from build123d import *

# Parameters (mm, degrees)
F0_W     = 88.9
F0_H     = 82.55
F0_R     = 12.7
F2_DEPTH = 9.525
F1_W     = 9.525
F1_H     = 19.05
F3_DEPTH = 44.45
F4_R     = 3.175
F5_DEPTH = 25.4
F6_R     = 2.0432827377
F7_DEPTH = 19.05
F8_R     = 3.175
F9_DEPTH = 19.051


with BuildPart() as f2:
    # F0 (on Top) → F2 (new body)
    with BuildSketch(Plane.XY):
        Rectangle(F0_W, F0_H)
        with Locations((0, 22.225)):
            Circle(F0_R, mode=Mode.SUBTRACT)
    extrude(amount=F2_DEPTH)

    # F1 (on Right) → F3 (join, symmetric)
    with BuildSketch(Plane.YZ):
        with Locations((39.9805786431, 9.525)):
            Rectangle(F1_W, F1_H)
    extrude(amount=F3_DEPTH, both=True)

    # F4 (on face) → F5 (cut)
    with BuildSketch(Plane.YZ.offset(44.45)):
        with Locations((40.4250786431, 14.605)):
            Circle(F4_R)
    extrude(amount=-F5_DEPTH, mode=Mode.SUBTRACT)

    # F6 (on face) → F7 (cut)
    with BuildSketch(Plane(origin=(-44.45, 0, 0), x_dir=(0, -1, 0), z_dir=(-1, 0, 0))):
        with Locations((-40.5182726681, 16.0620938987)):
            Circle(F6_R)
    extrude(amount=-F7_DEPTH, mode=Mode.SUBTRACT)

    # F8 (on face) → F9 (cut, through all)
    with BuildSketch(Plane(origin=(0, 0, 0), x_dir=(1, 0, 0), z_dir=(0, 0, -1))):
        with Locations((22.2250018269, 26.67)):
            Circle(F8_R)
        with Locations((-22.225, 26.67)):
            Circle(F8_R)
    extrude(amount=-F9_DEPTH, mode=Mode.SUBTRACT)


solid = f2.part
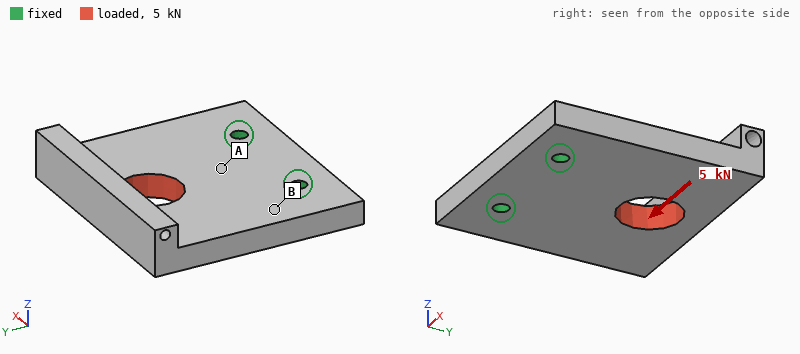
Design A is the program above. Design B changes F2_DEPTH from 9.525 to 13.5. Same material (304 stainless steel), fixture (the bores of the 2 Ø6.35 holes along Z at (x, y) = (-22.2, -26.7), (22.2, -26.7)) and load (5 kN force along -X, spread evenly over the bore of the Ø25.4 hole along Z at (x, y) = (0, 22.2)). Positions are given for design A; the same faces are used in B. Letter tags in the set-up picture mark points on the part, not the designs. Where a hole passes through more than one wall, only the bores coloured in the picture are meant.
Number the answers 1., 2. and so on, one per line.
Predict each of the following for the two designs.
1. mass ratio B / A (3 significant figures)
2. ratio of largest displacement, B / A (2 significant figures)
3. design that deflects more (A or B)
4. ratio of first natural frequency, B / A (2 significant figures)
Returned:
1. 1.33
2. 0.71
3. A
4. 1.5
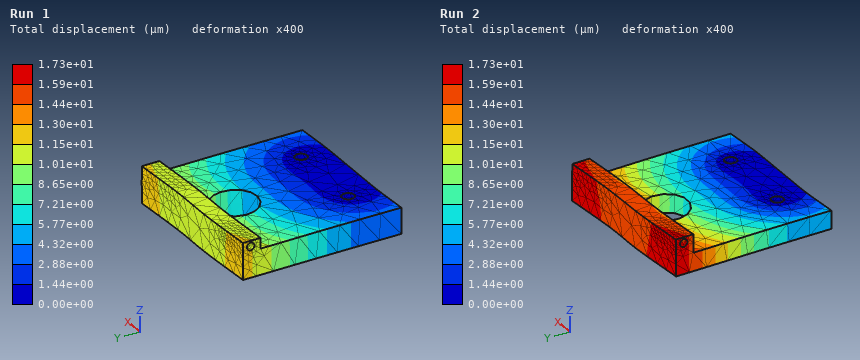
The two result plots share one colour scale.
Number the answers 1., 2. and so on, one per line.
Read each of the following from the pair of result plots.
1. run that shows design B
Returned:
1. Run 1
